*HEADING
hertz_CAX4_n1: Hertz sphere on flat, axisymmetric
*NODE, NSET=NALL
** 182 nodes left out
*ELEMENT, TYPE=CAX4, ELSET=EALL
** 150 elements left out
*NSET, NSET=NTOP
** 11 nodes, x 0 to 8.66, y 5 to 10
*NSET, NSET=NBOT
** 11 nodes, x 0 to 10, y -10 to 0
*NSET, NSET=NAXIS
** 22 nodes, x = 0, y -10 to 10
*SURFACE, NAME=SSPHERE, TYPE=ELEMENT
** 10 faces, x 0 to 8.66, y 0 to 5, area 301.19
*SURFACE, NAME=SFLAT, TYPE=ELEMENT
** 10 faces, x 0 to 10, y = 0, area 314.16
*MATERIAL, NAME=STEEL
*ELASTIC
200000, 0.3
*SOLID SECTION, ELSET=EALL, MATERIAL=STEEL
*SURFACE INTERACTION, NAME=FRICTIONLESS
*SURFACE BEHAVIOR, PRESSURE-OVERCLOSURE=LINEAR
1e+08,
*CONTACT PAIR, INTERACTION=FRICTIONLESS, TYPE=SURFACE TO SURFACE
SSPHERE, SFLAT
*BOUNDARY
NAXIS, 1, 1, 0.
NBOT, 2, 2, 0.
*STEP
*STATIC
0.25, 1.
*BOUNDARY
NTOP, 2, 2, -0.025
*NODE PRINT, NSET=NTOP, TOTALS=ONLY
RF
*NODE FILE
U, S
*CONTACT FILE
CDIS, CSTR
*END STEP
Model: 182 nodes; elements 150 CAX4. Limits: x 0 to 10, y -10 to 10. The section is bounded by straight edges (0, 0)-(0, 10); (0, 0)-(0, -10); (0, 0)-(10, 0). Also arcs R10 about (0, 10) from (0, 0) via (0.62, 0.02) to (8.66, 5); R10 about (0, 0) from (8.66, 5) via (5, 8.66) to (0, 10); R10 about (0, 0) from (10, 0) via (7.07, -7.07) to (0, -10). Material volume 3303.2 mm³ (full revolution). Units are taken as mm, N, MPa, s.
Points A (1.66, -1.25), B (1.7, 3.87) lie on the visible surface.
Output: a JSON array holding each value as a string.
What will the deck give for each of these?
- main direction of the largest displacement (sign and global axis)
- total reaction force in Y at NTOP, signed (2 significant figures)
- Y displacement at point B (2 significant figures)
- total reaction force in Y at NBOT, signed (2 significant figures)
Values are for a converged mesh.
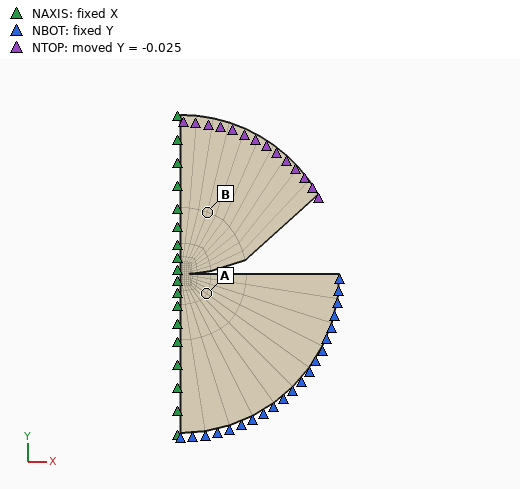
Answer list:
["-Y", "-1900 N", "-0.024 mm", "1900 N"]
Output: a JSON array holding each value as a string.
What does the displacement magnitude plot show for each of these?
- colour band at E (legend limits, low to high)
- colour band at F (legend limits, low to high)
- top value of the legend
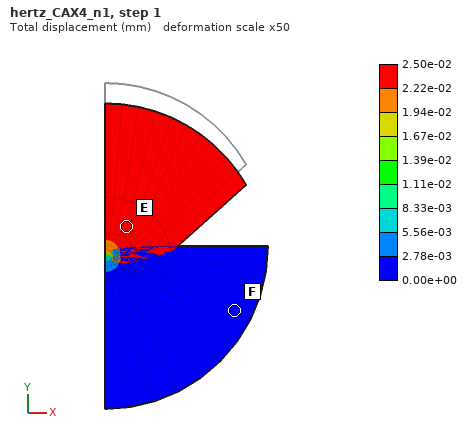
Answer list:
["2.22e-02 to 2.50e-02 mm", "0.00e+00 to 2.78e-03 mm", "2.50e-02 mm"]
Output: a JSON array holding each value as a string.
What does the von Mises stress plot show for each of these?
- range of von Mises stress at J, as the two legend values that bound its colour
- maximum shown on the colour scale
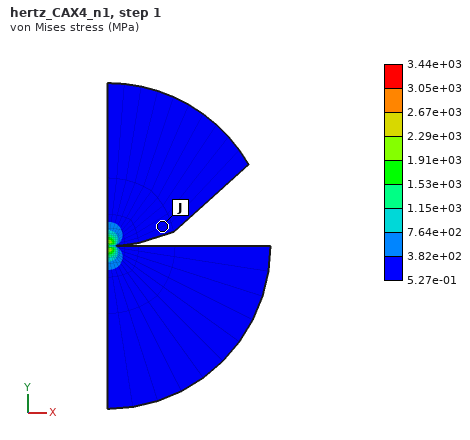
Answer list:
["5.27e-01 to 3.82e+02 MPa", "3.44e+03 MPa"]
